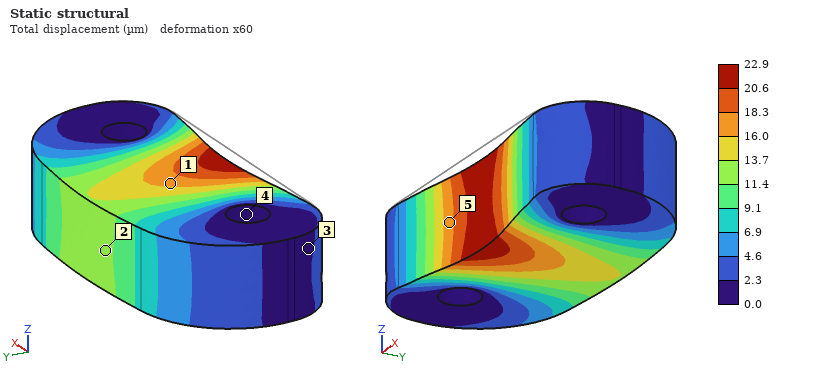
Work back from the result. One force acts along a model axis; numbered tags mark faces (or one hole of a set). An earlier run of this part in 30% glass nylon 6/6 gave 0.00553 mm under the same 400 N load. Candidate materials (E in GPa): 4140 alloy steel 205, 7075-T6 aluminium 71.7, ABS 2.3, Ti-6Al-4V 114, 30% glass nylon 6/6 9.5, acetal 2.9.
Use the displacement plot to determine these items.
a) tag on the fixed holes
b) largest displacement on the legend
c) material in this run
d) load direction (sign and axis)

4
22.9 µm
ABS
+Y
